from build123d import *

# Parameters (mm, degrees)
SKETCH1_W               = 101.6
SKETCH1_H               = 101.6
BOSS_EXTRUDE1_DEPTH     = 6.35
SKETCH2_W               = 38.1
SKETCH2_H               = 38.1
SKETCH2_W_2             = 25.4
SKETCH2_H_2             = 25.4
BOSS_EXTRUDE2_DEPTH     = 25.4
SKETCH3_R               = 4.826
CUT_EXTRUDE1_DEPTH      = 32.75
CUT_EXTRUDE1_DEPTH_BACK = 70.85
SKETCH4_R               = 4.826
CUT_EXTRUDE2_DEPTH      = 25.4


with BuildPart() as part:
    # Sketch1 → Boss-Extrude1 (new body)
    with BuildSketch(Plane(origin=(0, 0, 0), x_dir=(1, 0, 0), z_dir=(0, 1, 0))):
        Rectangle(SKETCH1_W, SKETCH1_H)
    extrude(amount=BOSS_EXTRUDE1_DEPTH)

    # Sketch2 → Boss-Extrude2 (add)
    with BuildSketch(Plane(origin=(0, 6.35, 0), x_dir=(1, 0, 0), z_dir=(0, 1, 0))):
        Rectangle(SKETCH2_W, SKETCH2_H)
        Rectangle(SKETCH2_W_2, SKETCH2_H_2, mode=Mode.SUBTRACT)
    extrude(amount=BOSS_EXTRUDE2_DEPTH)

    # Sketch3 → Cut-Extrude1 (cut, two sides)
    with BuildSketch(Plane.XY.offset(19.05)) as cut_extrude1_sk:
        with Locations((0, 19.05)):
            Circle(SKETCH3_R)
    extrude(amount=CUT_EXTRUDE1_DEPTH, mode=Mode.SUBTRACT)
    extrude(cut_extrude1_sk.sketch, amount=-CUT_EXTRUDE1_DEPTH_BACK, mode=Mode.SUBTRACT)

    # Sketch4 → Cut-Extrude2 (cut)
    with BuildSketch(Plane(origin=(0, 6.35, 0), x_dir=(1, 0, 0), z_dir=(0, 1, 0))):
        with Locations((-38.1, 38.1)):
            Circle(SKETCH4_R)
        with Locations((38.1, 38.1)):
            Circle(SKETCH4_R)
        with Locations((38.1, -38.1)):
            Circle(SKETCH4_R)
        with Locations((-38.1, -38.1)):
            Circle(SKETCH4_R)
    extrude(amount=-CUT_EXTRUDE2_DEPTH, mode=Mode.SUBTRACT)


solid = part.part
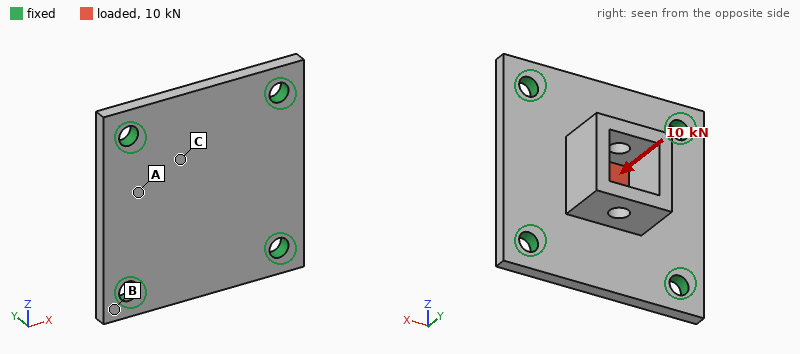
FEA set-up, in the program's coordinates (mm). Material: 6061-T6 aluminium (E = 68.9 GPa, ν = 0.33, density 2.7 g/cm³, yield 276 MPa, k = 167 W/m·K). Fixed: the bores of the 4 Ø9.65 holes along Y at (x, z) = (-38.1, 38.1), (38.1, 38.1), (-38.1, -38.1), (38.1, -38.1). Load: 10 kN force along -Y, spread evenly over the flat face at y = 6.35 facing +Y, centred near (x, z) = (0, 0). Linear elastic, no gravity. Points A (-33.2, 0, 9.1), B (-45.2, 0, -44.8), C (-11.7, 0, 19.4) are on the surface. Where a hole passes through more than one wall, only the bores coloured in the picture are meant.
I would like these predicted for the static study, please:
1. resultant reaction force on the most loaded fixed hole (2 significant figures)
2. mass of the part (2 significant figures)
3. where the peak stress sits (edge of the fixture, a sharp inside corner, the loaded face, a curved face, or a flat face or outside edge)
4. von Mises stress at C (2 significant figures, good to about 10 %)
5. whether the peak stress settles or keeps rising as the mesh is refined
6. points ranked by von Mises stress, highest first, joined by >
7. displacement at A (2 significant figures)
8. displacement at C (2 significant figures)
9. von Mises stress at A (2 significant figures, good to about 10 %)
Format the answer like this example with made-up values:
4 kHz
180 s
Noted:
2.6 kN
220 g
edge of the fixture
79 MPa
keeps rising
C > A > B
0.091 mm
0.14 mm
41 MPa
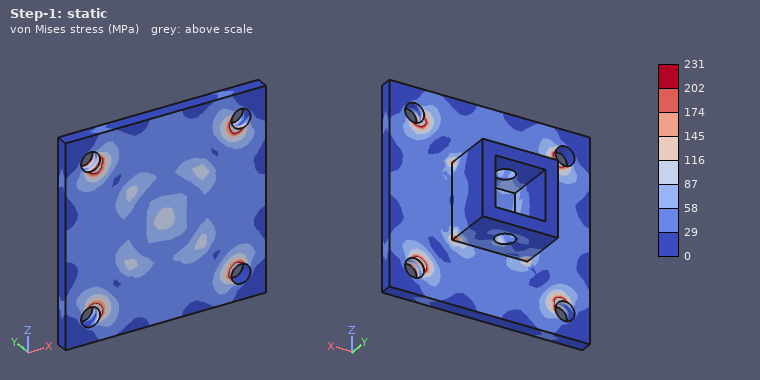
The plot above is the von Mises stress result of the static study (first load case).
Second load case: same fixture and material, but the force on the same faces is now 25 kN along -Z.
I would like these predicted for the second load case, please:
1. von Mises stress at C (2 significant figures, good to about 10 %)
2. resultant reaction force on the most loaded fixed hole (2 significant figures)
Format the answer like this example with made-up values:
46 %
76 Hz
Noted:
33 MPa
7.0 kN
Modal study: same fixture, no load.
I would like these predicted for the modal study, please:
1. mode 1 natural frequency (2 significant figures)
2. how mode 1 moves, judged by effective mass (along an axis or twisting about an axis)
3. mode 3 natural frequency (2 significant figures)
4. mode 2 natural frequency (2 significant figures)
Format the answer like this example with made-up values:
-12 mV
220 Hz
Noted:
3900 Hz
along Y
5600 Hz
5500 Hz
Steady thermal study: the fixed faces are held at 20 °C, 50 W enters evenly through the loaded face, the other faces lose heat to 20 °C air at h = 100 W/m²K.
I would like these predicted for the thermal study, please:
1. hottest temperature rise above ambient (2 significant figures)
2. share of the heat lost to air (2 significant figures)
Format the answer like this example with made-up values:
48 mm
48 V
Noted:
14 K
27 %
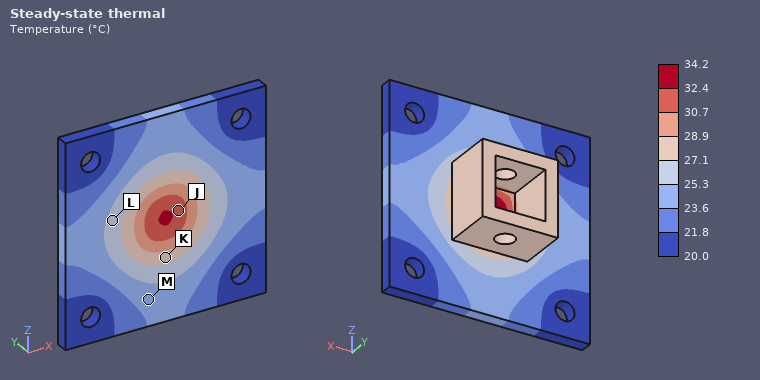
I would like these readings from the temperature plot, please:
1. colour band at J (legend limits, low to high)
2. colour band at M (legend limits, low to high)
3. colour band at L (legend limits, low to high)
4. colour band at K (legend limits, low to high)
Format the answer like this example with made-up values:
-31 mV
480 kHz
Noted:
30.7 to 32.4 °C
23.6 to 25.3 °C
25.3 to 27.1 °C
27.1 to 28.9 °C
